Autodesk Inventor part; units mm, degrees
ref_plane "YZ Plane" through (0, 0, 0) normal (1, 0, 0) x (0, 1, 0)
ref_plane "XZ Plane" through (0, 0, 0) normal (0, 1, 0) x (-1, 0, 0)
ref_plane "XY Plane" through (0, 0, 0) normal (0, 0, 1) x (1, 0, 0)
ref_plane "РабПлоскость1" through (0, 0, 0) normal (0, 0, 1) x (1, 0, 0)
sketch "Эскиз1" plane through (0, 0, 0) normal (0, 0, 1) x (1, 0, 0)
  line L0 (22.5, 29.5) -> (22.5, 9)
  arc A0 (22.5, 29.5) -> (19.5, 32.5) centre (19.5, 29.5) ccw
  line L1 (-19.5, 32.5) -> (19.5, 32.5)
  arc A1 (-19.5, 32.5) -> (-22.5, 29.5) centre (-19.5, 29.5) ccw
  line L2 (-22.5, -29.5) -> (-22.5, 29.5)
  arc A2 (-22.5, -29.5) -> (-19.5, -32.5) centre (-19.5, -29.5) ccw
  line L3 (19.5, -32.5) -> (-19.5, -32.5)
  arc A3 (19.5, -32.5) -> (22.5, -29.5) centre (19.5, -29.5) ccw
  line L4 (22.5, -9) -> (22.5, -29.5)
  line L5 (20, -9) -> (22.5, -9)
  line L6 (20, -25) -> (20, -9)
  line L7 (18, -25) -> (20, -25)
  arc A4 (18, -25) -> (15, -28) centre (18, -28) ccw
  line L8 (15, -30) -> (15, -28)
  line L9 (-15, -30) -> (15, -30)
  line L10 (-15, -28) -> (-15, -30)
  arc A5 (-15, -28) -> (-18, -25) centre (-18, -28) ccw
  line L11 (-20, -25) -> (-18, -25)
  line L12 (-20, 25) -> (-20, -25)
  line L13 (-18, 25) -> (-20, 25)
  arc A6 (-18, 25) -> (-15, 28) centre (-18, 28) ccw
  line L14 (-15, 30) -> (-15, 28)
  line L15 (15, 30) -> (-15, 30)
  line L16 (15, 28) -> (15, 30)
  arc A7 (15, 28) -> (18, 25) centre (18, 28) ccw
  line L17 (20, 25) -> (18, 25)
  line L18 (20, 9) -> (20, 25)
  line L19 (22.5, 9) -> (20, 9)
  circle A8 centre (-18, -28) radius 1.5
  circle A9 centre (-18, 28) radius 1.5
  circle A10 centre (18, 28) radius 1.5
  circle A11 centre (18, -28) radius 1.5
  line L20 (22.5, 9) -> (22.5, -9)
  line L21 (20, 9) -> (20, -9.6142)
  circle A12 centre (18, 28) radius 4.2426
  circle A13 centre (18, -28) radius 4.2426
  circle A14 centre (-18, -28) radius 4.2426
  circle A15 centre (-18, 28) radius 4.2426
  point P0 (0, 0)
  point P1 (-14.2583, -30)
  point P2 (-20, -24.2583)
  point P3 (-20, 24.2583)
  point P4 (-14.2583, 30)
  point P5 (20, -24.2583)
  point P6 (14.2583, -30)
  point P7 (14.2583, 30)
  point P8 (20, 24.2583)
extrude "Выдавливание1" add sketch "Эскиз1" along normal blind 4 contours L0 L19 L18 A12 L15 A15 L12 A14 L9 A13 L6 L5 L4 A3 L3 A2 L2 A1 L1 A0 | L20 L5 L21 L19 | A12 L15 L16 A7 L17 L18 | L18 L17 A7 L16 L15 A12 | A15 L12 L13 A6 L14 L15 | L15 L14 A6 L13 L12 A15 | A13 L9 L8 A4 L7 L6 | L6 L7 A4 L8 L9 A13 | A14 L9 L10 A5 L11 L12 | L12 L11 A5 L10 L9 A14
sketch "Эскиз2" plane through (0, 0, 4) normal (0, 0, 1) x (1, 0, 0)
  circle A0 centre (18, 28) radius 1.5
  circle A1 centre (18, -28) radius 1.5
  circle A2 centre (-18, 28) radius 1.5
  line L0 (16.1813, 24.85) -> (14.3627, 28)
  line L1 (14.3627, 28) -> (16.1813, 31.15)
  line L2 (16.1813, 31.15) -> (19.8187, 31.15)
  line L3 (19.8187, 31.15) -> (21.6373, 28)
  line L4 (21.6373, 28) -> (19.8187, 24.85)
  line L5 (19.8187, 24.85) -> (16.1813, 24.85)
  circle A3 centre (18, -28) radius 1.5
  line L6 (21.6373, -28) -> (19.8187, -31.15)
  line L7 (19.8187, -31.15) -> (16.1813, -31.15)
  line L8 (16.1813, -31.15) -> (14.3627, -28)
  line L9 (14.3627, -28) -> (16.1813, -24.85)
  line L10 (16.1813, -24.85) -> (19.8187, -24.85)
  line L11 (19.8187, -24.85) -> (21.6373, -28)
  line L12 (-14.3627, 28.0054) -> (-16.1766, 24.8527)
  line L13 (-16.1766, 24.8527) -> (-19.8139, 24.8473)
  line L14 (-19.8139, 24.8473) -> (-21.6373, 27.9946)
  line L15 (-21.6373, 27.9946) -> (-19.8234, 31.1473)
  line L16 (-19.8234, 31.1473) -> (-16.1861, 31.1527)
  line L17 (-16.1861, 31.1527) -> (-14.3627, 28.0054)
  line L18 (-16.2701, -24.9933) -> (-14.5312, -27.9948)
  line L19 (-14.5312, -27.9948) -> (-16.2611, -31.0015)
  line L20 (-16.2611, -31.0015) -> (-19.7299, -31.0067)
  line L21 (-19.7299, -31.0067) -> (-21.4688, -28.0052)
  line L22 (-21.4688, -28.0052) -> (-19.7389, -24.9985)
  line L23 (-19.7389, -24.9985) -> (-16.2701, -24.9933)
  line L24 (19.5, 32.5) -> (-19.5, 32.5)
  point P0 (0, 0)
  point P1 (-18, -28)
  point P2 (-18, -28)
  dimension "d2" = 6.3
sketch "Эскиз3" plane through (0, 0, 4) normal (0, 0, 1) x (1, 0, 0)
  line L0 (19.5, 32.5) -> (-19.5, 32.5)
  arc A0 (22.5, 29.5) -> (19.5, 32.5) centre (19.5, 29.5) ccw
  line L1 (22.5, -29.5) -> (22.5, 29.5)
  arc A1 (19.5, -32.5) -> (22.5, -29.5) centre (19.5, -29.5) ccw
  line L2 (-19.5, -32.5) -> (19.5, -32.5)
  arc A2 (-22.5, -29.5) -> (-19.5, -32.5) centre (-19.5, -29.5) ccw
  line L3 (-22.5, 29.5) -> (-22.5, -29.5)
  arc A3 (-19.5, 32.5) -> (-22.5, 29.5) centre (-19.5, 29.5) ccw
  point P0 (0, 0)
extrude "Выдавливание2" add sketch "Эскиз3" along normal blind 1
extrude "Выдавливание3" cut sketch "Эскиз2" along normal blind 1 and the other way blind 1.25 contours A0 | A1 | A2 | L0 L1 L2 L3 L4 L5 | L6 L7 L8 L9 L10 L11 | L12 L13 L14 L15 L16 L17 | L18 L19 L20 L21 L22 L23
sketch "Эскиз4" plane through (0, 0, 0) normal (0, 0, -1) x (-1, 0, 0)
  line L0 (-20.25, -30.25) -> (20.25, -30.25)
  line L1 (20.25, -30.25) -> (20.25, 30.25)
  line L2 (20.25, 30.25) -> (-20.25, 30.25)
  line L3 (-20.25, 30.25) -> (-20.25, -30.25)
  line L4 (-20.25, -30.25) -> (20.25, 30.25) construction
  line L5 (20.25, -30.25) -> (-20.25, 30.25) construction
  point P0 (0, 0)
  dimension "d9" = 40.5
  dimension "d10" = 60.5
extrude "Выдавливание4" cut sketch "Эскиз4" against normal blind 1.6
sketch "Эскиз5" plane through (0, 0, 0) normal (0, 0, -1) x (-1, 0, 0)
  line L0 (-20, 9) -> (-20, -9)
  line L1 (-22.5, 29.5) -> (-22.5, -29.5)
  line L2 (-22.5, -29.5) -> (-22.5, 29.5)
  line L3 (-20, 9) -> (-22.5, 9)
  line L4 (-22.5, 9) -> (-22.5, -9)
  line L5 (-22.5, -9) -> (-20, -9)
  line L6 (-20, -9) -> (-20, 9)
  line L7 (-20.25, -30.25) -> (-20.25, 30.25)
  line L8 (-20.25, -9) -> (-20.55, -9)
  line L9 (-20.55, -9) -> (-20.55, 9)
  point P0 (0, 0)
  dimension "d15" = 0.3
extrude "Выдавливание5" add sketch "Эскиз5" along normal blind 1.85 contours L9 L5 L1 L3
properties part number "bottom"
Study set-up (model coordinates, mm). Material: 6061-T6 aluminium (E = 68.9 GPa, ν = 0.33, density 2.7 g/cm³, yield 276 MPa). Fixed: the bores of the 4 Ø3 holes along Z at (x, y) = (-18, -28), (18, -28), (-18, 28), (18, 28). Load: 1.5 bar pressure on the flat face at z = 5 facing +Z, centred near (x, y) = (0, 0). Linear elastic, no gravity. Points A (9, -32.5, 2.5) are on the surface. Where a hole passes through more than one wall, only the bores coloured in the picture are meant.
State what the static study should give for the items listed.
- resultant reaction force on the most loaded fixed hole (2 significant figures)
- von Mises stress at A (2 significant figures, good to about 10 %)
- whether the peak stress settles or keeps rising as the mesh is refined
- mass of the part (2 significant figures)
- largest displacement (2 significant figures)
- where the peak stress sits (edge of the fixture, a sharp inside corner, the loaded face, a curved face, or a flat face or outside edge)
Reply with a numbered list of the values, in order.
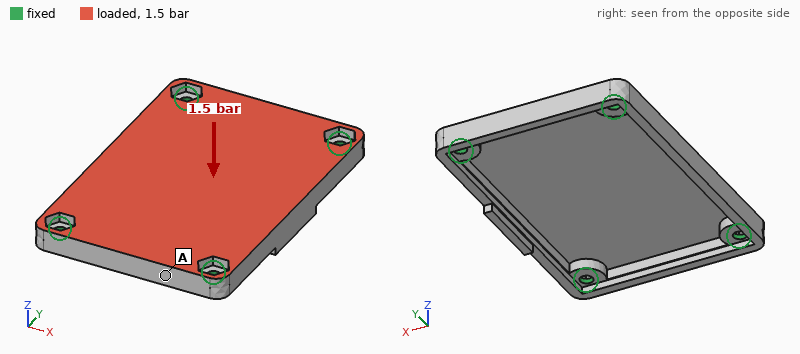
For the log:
1. 200 N
2. 15 MPa
3. keeps rising
4. 13 g
5. 0.24 mm
6. edge of the fixture
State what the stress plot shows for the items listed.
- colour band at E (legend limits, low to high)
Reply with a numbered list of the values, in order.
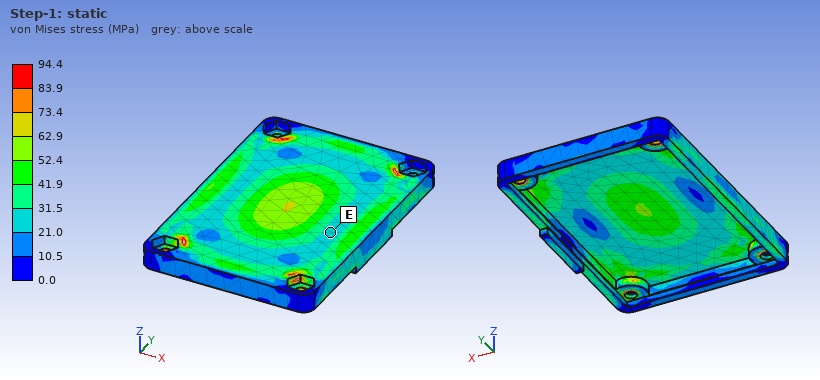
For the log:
1. 21.0 to 31.5 MPa
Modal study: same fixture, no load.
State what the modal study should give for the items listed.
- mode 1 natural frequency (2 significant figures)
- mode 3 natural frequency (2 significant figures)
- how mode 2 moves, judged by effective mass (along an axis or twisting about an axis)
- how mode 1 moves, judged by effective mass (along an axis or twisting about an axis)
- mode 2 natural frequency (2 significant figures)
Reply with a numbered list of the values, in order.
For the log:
1. 3100 Hz
2. 5700 Hz
3. twisting about Y
4. along Z
5. 5300 Hz
